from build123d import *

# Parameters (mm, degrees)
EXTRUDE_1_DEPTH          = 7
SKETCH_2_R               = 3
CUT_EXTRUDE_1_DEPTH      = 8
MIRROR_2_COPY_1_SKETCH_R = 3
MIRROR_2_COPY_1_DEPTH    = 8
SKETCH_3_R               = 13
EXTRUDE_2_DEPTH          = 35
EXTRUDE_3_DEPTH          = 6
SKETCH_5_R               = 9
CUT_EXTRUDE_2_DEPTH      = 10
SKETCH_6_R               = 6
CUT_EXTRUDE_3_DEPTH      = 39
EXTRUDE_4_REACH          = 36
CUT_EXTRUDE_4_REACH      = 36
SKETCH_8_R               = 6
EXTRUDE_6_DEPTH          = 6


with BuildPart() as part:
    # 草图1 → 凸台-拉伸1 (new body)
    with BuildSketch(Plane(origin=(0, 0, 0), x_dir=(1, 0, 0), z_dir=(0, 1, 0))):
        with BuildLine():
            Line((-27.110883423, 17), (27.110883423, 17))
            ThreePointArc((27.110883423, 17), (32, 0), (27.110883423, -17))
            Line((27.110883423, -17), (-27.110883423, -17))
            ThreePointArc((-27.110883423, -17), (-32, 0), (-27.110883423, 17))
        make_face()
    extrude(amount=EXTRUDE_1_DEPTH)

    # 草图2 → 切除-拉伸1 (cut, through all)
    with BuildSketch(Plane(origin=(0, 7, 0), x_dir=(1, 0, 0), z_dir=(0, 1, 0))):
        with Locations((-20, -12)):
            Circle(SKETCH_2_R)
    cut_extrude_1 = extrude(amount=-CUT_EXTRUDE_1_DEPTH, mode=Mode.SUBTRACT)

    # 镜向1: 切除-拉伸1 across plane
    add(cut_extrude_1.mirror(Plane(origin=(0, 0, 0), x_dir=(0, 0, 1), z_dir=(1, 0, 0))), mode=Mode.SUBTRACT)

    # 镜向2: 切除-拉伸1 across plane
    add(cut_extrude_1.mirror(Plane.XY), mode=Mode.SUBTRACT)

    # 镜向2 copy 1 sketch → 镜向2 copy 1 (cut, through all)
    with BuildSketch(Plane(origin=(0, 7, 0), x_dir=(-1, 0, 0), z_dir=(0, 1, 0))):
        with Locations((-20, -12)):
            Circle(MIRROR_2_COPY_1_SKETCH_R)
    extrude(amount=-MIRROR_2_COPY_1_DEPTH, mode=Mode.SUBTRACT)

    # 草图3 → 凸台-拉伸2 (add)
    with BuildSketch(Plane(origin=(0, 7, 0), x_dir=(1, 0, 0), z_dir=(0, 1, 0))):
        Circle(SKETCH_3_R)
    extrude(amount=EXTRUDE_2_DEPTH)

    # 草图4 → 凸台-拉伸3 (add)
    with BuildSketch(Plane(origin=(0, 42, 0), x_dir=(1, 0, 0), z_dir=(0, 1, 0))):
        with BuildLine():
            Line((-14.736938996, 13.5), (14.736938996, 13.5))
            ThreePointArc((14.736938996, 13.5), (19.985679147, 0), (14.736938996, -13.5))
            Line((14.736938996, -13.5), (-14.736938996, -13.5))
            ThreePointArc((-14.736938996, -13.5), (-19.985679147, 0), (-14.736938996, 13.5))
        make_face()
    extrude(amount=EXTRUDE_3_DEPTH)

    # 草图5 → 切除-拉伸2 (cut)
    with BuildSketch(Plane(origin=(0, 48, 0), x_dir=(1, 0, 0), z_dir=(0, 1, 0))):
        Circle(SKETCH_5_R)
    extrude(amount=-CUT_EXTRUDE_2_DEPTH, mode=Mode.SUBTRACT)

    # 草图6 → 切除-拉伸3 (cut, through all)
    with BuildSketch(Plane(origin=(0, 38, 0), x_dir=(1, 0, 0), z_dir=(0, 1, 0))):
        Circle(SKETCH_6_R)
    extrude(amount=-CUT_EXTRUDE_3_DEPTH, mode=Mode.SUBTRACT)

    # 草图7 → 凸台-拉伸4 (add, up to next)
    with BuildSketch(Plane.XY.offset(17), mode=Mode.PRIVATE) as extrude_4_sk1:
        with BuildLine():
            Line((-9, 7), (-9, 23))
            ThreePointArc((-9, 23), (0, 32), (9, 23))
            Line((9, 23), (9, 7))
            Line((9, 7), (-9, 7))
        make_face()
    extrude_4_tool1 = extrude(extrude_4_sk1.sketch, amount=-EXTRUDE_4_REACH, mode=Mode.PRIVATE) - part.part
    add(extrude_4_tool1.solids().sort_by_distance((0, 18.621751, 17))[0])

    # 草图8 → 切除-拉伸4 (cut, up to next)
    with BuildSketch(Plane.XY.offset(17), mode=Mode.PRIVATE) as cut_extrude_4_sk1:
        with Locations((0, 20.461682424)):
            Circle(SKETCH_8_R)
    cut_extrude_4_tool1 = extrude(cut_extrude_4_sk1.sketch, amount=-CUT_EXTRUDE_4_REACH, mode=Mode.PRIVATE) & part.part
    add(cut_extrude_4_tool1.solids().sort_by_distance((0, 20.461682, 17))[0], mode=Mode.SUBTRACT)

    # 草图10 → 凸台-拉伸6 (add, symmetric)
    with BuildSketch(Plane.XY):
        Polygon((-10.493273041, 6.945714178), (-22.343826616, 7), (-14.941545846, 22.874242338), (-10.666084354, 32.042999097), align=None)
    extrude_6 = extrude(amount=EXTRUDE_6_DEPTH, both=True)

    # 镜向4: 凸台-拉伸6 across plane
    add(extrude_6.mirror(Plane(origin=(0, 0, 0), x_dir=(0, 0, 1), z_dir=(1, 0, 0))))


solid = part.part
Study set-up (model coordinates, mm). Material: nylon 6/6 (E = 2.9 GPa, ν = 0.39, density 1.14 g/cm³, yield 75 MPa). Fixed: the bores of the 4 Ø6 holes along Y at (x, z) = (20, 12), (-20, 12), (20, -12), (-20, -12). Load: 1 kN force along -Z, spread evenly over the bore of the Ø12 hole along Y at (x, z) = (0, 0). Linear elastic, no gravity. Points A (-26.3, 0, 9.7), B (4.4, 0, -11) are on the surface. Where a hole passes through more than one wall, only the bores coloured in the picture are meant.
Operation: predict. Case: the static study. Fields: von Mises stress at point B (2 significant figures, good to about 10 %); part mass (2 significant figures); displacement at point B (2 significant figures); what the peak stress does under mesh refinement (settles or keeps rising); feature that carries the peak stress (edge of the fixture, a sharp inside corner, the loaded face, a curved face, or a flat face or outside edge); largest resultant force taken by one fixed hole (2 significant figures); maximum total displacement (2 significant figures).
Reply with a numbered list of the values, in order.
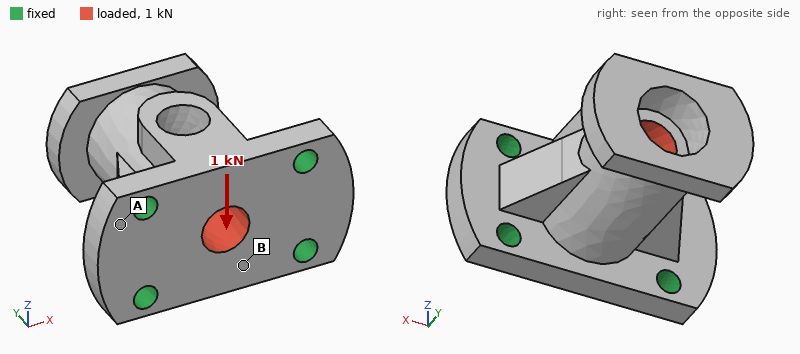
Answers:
1. 4.3 MPa
2. 39 g
3. 0.055 mm
4. keeps rising
5. edge of the fixture
6. 470 N
7. 0.32 mm
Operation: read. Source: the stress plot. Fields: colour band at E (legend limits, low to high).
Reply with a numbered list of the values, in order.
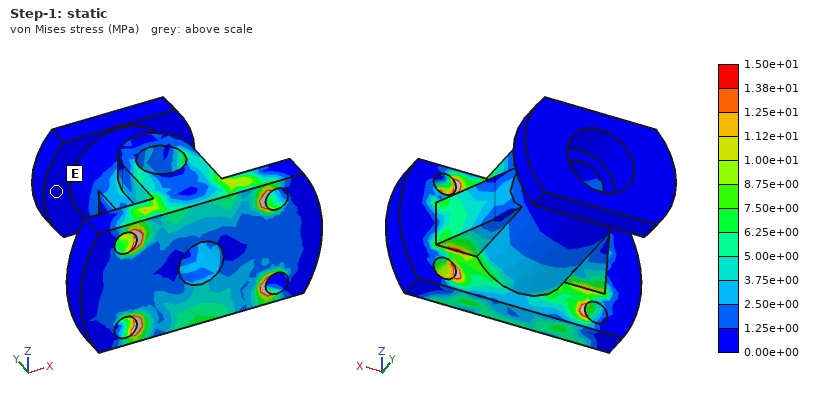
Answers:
1. 0.00e+00 to 1.25e+00 MPa
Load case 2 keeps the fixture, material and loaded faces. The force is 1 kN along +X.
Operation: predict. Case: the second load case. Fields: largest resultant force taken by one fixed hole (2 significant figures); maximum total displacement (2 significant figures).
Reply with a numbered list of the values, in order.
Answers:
1. 330 N
2. 0.10 mm
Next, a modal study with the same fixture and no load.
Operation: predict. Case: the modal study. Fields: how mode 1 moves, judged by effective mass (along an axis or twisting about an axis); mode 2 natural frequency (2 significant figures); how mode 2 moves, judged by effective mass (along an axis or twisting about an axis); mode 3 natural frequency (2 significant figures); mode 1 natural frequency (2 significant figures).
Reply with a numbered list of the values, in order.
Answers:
1. along Z
2. 2700 Hz
3. along X
4. 4300 Hz
5. 1700 Hz
